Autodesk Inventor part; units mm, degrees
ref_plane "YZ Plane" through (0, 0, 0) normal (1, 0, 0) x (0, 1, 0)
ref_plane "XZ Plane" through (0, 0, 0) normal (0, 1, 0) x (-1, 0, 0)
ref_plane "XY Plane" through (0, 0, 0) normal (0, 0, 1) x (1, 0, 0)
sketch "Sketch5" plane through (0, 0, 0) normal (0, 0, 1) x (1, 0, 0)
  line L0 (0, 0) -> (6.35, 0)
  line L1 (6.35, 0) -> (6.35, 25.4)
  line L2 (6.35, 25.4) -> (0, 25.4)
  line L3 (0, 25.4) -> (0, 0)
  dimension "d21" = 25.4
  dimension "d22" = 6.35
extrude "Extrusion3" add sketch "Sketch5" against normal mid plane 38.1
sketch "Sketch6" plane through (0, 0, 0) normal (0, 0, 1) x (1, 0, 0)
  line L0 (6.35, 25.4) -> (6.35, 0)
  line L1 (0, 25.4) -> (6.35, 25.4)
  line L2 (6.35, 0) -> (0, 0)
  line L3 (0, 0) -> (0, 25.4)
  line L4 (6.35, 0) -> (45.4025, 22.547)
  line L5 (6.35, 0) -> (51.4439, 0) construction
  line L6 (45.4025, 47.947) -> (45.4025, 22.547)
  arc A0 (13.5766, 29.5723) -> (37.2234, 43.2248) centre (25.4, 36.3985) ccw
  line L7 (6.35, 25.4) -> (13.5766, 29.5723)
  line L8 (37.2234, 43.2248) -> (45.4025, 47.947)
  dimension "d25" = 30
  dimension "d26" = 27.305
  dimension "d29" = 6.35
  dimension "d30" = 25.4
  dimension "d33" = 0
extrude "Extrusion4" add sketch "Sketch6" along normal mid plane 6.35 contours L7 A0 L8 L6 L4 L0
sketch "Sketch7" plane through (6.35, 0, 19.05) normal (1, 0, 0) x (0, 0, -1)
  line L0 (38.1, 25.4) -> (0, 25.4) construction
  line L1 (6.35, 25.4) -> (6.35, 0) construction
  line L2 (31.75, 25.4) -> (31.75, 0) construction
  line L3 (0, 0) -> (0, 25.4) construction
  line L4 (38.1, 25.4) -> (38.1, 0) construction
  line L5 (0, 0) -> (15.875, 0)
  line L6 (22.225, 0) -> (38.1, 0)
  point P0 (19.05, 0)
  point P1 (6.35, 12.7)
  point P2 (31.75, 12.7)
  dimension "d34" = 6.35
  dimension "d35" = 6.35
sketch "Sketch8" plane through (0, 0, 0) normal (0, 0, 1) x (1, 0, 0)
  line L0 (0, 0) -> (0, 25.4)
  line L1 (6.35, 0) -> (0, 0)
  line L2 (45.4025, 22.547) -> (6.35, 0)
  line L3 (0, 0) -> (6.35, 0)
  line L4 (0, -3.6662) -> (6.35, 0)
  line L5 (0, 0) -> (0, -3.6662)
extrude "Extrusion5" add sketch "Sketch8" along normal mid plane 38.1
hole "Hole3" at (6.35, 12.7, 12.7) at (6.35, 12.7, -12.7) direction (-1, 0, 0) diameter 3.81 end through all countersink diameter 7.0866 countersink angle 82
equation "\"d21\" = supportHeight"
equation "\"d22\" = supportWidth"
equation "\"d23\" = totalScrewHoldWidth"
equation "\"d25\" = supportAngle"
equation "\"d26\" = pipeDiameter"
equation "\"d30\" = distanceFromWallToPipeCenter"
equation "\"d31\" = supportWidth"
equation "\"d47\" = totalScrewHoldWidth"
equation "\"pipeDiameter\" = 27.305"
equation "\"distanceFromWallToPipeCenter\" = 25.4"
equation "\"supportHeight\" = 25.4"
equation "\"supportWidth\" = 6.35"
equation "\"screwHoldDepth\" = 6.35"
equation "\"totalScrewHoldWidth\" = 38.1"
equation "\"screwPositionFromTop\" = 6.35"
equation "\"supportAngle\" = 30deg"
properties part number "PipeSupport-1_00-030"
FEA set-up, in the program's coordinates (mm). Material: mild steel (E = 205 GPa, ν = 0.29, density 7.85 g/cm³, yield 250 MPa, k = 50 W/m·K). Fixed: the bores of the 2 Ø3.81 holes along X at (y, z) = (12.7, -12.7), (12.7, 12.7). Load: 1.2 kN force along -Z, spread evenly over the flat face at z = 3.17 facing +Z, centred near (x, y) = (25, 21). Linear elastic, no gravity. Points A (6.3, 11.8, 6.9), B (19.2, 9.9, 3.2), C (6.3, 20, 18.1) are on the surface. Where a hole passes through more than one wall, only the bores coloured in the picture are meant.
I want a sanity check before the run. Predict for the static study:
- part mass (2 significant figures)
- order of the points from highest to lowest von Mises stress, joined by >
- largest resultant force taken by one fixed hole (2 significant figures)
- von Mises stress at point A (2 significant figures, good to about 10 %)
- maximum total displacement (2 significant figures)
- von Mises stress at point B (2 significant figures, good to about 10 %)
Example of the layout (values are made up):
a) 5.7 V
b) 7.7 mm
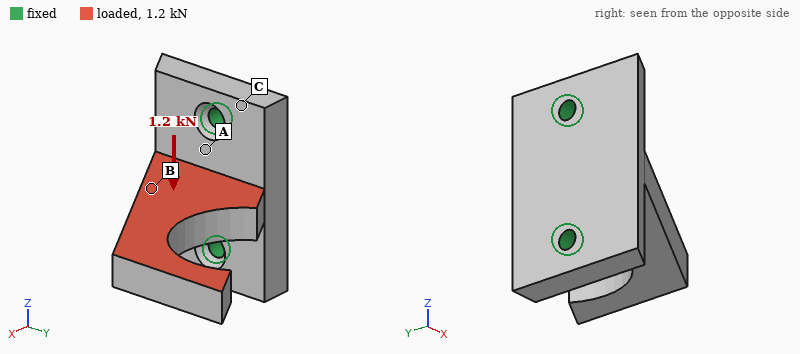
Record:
a) 85 g
b) B > A > C
c) 1.4 kN
d) 34 MPa
e) 0.25 mm
f) 110 MPa
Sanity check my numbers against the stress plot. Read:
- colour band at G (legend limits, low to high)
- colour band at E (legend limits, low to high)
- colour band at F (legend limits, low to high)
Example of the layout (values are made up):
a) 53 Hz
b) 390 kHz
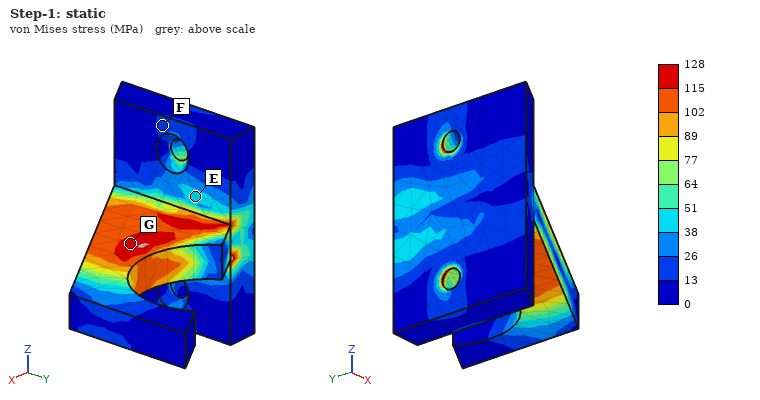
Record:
a) 115 to 128 MPa
b) 38 to 51 MPa
c) 13 to 26 MPa
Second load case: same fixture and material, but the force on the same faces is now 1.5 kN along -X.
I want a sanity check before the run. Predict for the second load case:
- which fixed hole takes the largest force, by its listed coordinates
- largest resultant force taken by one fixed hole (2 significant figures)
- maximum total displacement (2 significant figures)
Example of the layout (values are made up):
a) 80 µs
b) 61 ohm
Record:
a) (12.7, 12.7)
b) 1.0 kN
c) 0.10 mm
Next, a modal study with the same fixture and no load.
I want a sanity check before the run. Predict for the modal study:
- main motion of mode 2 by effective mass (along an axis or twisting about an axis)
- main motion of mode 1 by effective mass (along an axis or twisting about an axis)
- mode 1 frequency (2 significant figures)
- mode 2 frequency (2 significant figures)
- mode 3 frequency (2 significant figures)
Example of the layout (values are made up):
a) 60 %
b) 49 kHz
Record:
a) along Y
b) along Z
c) 2400 Hz
d) 3300 Hz
e) 7300 Hz
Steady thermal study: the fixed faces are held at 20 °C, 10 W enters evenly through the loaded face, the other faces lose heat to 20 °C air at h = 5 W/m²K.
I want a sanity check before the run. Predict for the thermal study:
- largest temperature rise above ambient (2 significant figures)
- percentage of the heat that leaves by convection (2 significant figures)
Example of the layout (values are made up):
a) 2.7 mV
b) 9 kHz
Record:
a) 59 K
b) 3.4 %
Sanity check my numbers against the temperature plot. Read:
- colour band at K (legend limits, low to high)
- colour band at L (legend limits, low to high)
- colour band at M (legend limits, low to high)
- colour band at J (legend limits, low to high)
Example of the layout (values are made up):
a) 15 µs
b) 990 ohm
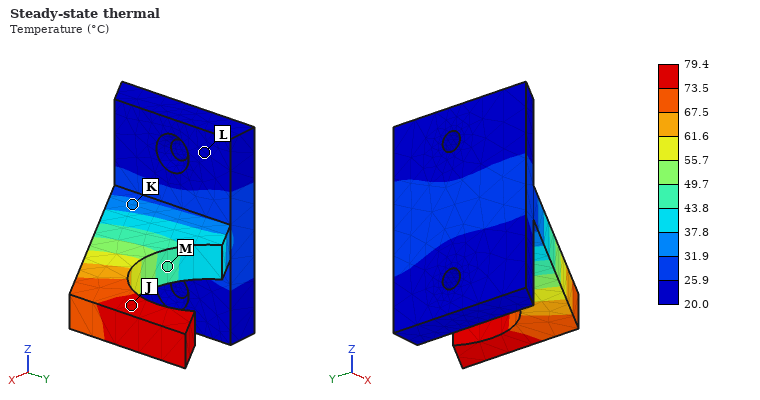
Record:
a) 31.9 to 37.8 °C
b) 20.0 to 25.9 °C
c) 43.8 to 49.7 °C
d) 73.5 to 79.4 °C
